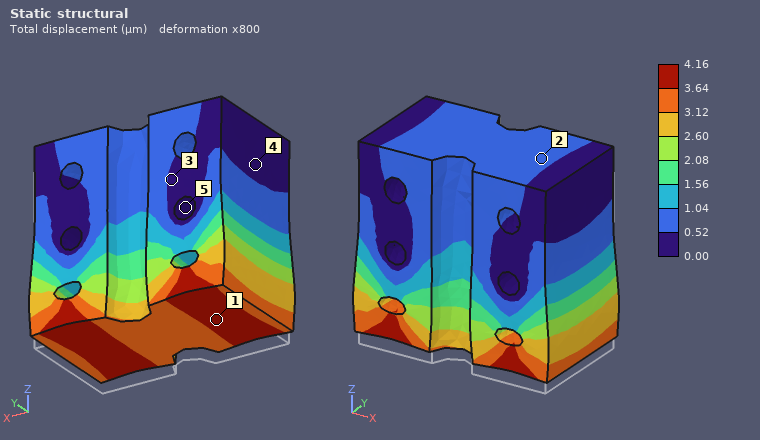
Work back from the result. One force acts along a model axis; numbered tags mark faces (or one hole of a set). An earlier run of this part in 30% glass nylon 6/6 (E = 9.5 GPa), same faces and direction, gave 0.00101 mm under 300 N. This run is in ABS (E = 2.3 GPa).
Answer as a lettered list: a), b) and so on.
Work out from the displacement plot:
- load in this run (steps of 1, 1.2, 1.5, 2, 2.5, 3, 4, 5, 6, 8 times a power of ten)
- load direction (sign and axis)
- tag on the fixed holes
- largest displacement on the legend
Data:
a) 300 N
b) +Z
c) 5
d) 4.16 µm
